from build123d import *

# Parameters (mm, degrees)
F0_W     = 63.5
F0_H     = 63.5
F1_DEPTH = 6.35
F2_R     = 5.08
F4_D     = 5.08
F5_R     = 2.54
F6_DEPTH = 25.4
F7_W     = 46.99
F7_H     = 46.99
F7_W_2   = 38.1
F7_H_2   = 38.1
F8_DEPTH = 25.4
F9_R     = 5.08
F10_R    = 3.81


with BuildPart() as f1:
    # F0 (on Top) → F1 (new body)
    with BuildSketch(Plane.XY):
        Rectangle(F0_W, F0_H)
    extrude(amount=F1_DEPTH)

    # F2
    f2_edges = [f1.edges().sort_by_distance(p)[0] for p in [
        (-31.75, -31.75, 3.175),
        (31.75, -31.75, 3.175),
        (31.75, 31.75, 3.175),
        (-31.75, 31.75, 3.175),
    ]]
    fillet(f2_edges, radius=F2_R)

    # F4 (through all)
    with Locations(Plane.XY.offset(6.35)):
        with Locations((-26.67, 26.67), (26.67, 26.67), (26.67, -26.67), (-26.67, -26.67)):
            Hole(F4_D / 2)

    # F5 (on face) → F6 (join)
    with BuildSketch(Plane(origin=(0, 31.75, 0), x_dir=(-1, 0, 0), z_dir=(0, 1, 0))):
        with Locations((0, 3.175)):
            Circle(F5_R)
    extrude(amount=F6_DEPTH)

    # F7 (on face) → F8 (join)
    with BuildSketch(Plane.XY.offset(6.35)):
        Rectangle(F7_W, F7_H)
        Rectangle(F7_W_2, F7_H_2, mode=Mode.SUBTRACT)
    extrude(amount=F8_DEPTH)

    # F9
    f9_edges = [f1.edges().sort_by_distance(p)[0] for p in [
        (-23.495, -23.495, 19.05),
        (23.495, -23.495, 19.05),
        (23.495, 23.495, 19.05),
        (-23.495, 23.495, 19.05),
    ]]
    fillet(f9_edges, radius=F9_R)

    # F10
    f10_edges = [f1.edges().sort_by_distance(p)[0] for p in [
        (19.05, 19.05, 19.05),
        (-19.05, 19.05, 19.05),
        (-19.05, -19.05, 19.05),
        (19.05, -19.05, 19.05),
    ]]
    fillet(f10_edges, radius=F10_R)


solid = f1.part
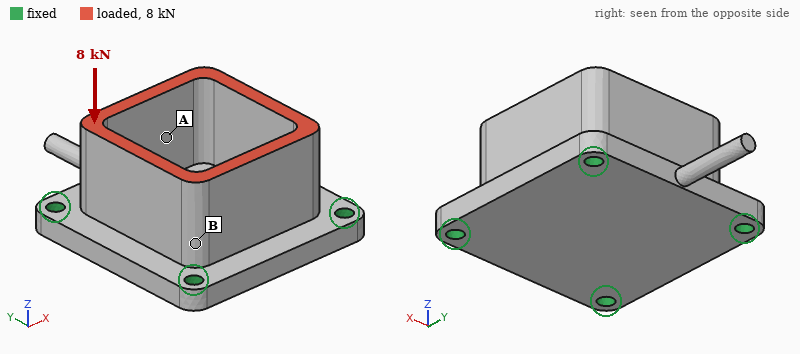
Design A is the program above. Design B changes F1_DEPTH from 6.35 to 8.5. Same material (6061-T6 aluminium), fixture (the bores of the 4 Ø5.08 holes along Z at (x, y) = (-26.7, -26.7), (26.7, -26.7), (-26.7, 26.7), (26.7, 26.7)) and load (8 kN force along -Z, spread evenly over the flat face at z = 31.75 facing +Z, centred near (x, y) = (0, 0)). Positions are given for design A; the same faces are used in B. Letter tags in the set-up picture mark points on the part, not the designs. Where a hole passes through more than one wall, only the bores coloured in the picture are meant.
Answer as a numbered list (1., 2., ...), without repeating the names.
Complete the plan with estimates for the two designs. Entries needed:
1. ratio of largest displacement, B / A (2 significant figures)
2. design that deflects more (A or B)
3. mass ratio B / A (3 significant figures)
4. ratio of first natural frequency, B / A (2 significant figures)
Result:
1. 0.68
2. A
3. 1.15
4. 1.1
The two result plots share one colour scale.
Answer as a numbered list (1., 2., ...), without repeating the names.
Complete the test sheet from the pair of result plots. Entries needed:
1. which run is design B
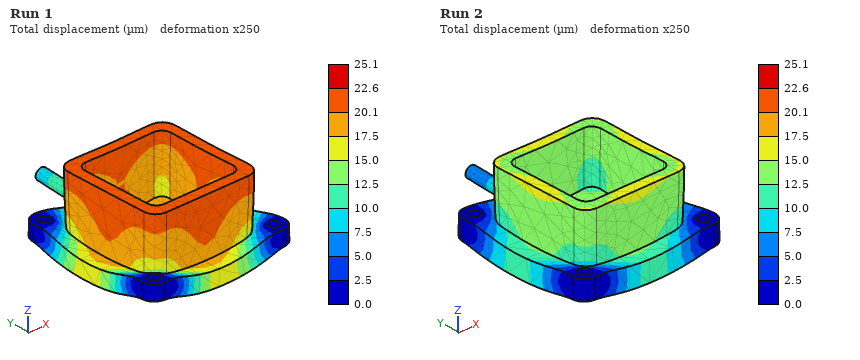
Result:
1. Run 2
